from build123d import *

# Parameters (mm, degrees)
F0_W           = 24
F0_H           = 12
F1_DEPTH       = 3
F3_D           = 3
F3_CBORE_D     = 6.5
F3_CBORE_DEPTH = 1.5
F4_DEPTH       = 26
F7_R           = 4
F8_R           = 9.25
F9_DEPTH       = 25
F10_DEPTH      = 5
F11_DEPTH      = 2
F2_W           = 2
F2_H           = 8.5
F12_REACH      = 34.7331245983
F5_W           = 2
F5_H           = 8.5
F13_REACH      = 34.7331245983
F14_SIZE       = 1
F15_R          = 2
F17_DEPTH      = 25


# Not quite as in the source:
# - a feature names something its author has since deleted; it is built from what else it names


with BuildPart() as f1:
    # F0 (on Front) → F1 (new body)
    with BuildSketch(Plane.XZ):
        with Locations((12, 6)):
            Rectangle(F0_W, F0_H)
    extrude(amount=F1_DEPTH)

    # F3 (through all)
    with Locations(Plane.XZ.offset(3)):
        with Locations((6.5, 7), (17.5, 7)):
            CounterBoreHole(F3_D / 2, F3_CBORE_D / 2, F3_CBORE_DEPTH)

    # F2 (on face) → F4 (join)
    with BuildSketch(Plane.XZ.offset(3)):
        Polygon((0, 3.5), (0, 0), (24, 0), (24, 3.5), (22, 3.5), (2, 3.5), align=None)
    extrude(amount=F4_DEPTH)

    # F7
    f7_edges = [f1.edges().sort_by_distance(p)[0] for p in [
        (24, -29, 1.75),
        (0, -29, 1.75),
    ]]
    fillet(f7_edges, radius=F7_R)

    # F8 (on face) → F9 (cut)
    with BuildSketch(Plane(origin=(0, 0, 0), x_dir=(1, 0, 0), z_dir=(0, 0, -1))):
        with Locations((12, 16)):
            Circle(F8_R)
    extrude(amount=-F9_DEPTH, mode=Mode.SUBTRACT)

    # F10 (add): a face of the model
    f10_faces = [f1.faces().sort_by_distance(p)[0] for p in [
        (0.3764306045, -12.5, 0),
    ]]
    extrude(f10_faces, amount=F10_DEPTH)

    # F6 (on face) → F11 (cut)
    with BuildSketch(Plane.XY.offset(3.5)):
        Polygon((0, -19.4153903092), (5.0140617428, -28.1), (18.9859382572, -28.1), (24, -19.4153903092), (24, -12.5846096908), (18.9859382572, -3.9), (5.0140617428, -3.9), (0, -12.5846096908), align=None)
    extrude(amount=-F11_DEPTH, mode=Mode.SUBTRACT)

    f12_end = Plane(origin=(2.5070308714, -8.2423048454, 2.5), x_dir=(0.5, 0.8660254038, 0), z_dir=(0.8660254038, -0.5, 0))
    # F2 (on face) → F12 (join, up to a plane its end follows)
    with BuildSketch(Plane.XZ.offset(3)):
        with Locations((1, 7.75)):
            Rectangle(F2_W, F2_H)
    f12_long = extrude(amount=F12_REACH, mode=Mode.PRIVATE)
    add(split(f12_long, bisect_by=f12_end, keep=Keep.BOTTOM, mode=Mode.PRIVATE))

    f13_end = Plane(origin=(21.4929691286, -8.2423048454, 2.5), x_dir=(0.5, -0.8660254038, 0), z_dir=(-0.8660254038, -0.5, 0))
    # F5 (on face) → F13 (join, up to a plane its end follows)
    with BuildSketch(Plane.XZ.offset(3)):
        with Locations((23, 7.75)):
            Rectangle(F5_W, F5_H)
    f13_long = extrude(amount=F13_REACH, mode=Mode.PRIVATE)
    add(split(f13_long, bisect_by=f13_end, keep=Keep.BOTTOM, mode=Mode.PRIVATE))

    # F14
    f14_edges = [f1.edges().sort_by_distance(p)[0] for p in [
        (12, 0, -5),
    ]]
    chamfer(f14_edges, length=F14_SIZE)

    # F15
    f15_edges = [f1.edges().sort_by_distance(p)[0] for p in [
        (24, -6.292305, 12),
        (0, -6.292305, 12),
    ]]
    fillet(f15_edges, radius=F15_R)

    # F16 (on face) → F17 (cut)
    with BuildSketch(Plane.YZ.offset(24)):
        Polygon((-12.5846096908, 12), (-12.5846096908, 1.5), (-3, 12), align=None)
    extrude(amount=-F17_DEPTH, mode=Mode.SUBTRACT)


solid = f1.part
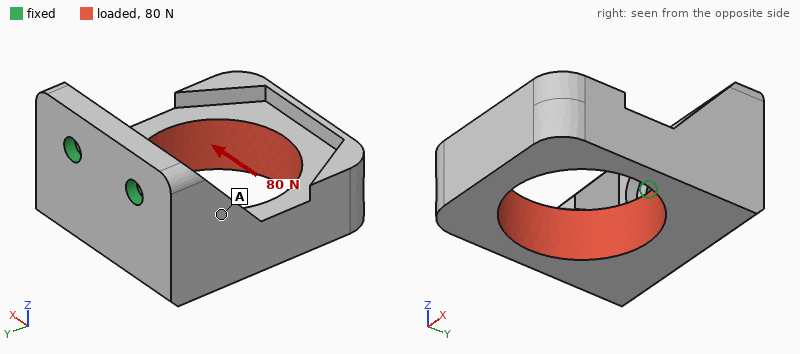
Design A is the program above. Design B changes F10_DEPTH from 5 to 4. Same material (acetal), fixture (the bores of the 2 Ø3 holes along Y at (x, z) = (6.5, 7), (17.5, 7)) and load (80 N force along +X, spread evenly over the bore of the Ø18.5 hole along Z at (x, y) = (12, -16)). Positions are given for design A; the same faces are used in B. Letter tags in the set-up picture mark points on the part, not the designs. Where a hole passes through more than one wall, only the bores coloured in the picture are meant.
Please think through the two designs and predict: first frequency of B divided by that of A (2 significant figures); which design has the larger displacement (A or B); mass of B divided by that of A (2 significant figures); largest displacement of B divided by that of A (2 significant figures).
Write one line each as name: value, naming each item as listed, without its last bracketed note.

first frequency of B divided by that of A: 1.1
which design has the larger displacement: B
mass of B divided by that of A: 0.89
largest displacement of B divided by that of A: 1.1
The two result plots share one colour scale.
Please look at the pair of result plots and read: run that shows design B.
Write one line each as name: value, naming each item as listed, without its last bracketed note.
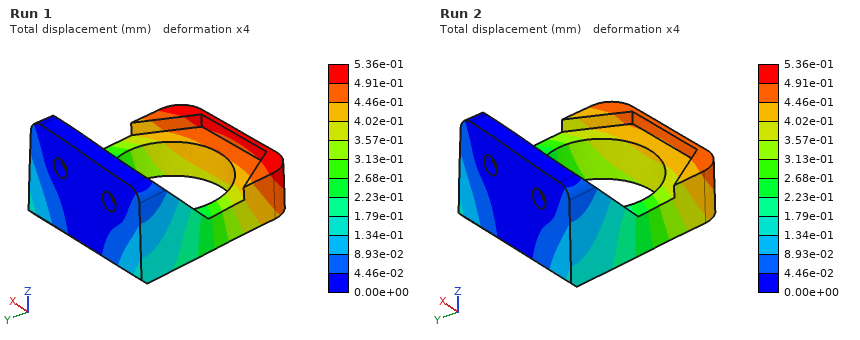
run that shows design B: Run 1
